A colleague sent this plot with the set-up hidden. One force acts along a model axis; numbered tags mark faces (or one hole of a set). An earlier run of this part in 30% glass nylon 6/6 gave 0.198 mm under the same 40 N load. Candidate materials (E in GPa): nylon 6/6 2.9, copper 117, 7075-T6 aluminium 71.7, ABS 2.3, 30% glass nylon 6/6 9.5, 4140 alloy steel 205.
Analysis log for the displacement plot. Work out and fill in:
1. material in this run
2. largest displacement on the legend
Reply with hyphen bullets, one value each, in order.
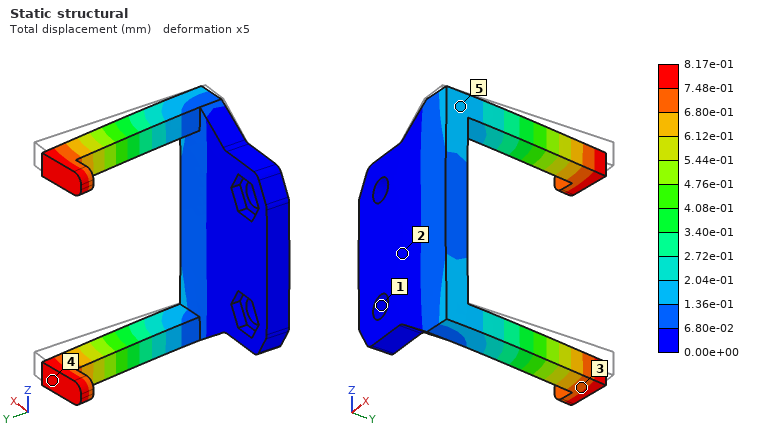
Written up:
- ABS
- 8.17e-01 mm
